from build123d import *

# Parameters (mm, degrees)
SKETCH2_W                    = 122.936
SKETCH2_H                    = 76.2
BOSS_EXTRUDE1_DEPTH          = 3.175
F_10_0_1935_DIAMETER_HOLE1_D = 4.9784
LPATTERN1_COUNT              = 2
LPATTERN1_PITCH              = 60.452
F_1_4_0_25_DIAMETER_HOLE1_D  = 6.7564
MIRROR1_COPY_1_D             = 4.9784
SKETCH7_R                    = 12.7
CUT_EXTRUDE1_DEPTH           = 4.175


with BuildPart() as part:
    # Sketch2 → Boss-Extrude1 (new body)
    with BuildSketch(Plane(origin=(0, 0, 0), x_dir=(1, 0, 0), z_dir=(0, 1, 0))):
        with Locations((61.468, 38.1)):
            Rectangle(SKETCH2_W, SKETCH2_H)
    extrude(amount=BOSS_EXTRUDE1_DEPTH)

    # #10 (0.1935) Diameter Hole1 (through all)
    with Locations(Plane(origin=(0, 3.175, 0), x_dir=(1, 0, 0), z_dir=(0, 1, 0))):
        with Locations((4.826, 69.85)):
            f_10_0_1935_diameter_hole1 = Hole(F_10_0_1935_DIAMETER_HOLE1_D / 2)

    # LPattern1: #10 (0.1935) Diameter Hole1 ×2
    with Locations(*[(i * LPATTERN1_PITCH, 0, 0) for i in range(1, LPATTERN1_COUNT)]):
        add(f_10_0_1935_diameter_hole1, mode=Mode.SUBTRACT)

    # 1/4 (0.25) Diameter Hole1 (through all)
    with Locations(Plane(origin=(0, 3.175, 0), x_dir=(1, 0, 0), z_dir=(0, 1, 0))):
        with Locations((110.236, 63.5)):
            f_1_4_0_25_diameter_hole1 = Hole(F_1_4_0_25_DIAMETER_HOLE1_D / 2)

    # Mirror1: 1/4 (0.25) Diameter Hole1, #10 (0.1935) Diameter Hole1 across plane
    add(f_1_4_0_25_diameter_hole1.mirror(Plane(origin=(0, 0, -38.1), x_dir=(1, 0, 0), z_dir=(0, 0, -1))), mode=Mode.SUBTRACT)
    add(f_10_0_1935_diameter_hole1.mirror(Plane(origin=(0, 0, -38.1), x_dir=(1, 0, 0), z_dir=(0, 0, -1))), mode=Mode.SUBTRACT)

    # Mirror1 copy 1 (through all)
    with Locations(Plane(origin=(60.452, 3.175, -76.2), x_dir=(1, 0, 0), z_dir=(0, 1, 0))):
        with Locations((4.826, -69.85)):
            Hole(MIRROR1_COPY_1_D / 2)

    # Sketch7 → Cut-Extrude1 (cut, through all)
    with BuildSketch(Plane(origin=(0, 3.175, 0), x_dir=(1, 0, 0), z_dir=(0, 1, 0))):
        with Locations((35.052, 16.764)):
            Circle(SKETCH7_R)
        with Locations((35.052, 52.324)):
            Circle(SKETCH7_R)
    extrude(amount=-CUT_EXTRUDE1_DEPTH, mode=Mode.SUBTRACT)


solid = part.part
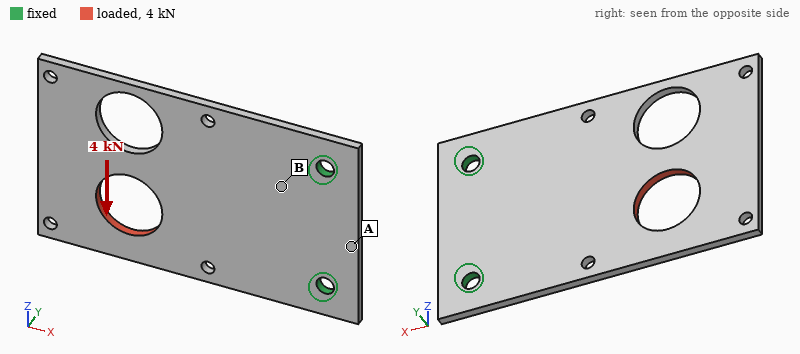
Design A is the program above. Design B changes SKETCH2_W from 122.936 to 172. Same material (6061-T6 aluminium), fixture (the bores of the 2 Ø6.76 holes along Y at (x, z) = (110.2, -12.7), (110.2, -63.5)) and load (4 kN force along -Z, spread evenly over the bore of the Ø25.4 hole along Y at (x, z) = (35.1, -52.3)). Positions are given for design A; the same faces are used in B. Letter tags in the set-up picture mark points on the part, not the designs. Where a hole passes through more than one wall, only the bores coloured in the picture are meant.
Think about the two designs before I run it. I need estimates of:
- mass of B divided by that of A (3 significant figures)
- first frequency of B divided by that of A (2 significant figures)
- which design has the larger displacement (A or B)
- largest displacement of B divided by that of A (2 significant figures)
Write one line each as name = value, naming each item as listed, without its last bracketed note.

mass of B divided by that of A = 1.46
first frequency of B divided by that of A = 0.62
which design has the larger displacement = B
largest displacement of B divided by that of A = 1.2
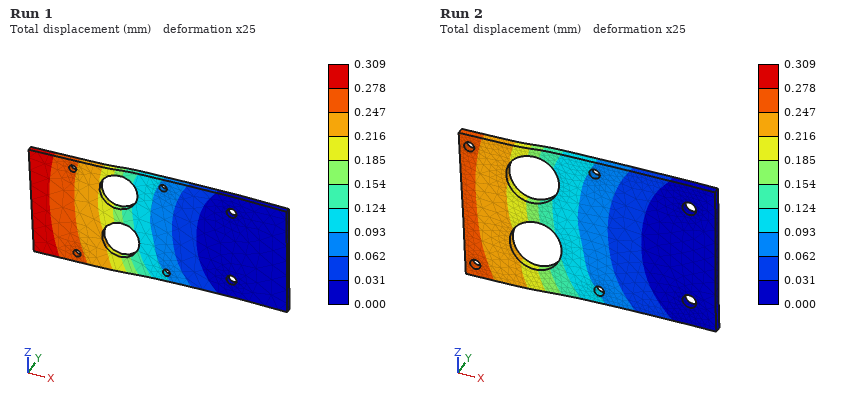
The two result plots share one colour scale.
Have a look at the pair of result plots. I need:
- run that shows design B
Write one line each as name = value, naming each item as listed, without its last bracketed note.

run that shows design B = Run 1
